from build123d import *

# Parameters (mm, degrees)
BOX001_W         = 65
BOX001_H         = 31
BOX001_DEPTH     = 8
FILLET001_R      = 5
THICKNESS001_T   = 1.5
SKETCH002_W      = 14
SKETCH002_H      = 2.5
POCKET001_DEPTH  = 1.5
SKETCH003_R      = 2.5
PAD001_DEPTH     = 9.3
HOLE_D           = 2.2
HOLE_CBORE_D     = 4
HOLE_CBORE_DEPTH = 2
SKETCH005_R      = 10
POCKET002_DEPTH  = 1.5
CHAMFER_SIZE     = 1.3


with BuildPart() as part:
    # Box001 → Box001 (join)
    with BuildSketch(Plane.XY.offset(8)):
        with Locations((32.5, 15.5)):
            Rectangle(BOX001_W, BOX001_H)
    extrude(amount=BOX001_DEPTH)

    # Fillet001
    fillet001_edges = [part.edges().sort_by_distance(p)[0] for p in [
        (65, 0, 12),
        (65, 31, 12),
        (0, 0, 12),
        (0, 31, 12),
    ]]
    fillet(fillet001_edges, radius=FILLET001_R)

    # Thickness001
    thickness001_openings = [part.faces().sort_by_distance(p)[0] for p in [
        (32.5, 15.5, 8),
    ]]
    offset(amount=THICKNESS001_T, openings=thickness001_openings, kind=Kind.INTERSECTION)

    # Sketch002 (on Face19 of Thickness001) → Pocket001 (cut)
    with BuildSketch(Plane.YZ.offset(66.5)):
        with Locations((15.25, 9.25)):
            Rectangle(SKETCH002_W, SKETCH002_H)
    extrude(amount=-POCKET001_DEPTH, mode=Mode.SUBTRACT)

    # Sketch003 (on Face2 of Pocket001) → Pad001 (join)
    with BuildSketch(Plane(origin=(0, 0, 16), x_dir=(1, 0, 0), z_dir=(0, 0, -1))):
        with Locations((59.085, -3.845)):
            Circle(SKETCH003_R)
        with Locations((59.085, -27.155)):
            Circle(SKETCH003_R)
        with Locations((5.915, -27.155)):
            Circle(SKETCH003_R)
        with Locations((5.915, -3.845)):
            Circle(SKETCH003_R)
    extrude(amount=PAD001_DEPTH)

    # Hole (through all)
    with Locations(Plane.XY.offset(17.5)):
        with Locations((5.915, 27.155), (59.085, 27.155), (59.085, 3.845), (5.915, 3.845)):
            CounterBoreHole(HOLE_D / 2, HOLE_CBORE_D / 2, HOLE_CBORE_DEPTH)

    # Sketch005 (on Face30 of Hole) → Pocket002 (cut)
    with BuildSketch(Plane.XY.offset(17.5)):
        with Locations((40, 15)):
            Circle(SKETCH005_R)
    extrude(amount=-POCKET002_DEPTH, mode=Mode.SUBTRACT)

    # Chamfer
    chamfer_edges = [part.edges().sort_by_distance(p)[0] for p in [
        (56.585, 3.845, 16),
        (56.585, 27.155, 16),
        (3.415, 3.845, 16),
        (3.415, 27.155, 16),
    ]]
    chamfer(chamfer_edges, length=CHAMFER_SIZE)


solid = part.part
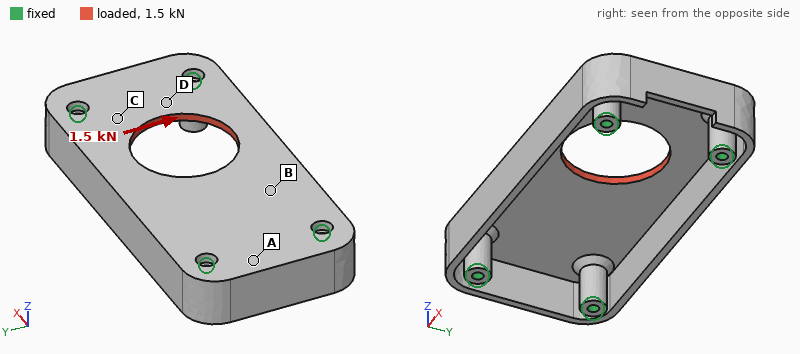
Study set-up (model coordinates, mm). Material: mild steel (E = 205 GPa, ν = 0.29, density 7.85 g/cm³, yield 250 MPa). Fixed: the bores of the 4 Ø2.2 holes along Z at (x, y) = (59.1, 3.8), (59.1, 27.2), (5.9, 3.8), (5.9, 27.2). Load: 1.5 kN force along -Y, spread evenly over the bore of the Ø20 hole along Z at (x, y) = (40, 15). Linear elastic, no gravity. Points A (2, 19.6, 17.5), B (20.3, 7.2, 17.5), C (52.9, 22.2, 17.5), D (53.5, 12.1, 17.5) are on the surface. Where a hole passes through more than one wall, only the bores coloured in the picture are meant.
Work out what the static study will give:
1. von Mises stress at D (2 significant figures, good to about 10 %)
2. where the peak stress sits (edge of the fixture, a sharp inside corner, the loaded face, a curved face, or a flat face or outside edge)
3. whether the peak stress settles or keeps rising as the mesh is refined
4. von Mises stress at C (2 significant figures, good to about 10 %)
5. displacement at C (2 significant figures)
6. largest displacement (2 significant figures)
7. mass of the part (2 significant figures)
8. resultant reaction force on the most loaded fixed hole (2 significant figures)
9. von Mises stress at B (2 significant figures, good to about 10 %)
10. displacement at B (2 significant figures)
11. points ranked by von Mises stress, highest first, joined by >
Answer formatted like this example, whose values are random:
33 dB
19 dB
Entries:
42 MPa
edge of the fixture
keeps rising
32 MPa
3.7 µm
10 µm
45 g
440 N
21 MPa
5.6 µm
D > C > B > A
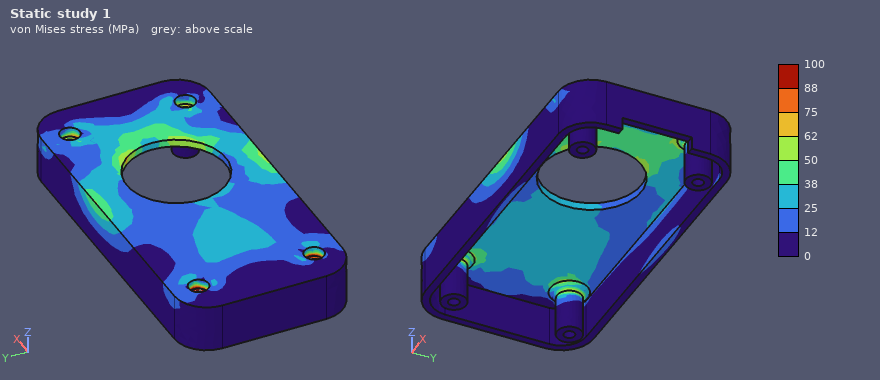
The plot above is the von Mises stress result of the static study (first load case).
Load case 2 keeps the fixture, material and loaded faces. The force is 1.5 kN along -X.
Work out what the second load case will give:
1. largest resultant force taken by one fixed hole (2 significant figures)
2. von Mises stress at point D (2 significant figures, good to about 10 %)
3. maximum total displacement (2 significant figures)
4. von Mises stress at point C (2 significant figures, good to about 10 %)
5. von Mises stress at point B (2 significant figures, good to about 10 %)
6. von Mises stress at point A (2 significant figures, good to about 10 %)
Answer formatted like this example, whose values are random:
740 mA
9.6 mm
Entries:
430 N
14 MPa
4.7 µm
19 MPa
14 MPa
9.1 MPa
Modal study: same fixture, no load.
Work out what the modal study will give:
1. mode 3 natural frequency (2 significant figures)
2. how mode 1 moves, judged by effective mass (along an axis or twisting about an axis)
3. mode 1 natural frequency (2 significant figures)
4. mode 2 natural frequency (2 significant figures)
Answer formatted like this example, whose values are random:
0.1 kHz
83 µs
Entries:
8000 Hz
along Z
5400 Hz
7900 Hz
